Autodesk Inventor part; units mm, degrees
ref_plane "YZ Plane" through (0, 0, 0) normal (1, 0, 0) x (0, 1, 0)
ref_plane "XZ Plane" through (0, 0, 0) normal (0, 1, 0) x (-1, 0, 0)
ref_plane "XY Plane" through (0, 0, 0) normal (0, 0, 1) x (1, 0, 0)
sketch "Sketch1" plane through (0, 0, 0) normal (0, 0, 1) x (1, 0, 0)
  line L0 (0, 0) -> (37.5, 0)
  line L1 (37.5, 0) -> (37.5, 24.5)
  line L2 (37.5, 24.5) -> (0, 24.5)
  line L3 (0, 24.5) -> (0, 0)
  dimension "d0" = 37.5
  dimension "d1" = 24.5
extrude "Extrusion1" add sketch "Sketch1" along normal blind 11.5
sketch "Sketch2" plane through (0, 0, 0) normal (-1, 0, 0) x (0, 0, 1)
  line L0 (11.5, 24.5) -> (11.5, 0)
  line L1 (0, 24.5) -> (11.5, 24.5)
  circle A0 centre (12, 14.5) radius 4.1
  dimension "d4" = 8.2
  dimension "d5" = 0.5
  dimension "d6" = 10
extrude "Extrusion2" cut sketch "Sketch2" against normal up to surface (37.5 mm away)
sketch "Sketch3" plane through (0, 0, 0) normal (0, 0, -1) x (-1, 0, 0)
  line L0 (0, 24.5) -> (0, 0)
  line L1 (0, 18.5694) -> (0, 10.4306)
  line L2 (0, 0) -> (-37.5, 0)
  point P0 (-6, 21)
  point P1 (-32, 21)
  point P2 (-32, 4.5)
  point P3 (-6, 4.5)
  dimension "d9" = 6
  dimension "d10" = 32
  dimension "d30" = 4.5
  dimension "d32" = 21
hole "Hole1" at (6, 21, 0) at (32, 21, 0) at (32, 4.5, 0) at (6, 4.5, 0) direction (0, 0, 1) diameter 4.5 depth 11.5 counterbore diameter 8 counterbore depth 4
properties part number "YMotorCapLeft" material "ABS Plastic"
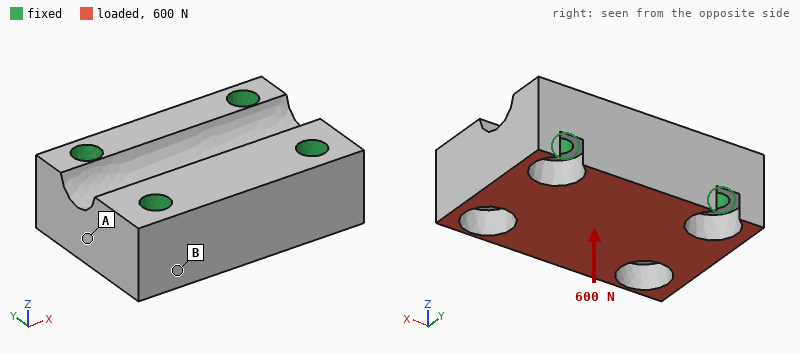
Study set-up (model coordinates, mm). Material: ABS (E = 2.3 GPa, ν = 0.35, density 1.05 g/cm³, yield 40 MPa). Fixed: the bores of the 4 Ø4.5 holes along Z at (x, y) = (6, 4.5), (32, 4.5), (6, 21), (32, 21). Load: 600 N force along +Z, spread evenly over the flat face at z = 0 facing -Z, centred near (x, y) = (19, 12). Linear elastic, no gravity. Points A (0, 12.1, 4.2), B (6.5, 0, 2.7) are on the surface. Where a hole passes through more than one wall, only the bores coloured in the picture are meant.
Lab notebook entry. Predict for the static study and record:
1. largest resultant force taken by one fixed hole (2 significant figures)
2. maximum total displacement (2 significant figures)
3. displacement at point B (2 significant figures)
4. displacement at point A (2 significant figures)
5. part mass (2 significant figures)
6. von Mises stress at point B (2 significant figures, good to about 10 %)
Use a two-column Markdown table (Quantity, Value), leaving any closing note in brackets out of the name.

| Quantity | Value |
|---|---|
| largest resultant force taken by one fixed hole | 170 N |
| maximum total displacement | 16 µm |
| displacement at point B | 3.4 µm |
| displacement at point A | 5.3 µm |
| part mass | 8.9 g |
| von Mises stress at point B | 1.5 MPa |
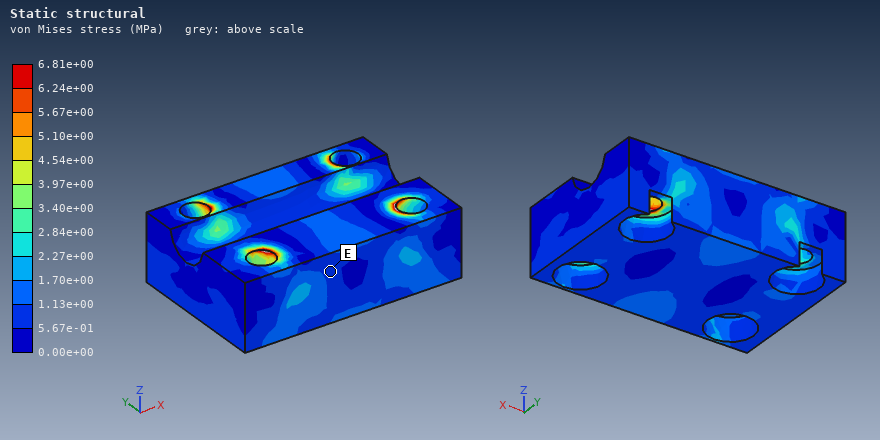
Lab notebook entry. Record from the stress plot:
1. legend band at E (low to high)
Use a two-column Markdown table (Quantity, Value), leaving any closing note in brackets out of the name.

| Quantity | Value |
|---|---|
| legend band at E | 5.67e-01 to 1.13e+00 MPa |
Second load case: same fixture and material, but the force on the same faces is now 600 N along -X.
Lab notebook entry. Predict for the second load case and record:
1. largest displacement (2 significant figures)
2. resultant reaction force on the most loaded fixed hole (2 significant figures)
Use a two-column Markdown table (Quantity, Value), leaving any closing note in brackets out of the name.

| Quantity | Value |
|---|---|
| largest displacement | 35 µm |
| resultant reaction force on the most loaded fixed hole | 180 N |
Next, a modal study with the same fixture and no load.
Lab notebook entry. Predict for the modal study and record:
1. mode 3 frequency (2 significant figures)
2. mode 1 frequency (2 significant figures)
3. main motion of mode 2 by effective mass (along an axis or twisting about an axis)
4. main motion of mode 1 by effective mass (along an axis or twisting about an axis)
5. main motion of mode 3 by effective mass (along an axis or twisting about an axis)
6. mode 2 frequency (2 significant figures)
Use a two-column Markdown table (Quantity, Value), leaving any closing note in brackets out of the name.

| Quantity | Value |
|---|---|
| mode 3 frequency | 15 kHz |
| mode 1 frequency | 12 kHz |
| main motion of mode 2 by effective mass | along Y |
| main motion of mode 1 by effective mass | along Z |
| main motion of mode 3 by effective mass | along Y |
| mode 2 frequency | 14 kHz |
